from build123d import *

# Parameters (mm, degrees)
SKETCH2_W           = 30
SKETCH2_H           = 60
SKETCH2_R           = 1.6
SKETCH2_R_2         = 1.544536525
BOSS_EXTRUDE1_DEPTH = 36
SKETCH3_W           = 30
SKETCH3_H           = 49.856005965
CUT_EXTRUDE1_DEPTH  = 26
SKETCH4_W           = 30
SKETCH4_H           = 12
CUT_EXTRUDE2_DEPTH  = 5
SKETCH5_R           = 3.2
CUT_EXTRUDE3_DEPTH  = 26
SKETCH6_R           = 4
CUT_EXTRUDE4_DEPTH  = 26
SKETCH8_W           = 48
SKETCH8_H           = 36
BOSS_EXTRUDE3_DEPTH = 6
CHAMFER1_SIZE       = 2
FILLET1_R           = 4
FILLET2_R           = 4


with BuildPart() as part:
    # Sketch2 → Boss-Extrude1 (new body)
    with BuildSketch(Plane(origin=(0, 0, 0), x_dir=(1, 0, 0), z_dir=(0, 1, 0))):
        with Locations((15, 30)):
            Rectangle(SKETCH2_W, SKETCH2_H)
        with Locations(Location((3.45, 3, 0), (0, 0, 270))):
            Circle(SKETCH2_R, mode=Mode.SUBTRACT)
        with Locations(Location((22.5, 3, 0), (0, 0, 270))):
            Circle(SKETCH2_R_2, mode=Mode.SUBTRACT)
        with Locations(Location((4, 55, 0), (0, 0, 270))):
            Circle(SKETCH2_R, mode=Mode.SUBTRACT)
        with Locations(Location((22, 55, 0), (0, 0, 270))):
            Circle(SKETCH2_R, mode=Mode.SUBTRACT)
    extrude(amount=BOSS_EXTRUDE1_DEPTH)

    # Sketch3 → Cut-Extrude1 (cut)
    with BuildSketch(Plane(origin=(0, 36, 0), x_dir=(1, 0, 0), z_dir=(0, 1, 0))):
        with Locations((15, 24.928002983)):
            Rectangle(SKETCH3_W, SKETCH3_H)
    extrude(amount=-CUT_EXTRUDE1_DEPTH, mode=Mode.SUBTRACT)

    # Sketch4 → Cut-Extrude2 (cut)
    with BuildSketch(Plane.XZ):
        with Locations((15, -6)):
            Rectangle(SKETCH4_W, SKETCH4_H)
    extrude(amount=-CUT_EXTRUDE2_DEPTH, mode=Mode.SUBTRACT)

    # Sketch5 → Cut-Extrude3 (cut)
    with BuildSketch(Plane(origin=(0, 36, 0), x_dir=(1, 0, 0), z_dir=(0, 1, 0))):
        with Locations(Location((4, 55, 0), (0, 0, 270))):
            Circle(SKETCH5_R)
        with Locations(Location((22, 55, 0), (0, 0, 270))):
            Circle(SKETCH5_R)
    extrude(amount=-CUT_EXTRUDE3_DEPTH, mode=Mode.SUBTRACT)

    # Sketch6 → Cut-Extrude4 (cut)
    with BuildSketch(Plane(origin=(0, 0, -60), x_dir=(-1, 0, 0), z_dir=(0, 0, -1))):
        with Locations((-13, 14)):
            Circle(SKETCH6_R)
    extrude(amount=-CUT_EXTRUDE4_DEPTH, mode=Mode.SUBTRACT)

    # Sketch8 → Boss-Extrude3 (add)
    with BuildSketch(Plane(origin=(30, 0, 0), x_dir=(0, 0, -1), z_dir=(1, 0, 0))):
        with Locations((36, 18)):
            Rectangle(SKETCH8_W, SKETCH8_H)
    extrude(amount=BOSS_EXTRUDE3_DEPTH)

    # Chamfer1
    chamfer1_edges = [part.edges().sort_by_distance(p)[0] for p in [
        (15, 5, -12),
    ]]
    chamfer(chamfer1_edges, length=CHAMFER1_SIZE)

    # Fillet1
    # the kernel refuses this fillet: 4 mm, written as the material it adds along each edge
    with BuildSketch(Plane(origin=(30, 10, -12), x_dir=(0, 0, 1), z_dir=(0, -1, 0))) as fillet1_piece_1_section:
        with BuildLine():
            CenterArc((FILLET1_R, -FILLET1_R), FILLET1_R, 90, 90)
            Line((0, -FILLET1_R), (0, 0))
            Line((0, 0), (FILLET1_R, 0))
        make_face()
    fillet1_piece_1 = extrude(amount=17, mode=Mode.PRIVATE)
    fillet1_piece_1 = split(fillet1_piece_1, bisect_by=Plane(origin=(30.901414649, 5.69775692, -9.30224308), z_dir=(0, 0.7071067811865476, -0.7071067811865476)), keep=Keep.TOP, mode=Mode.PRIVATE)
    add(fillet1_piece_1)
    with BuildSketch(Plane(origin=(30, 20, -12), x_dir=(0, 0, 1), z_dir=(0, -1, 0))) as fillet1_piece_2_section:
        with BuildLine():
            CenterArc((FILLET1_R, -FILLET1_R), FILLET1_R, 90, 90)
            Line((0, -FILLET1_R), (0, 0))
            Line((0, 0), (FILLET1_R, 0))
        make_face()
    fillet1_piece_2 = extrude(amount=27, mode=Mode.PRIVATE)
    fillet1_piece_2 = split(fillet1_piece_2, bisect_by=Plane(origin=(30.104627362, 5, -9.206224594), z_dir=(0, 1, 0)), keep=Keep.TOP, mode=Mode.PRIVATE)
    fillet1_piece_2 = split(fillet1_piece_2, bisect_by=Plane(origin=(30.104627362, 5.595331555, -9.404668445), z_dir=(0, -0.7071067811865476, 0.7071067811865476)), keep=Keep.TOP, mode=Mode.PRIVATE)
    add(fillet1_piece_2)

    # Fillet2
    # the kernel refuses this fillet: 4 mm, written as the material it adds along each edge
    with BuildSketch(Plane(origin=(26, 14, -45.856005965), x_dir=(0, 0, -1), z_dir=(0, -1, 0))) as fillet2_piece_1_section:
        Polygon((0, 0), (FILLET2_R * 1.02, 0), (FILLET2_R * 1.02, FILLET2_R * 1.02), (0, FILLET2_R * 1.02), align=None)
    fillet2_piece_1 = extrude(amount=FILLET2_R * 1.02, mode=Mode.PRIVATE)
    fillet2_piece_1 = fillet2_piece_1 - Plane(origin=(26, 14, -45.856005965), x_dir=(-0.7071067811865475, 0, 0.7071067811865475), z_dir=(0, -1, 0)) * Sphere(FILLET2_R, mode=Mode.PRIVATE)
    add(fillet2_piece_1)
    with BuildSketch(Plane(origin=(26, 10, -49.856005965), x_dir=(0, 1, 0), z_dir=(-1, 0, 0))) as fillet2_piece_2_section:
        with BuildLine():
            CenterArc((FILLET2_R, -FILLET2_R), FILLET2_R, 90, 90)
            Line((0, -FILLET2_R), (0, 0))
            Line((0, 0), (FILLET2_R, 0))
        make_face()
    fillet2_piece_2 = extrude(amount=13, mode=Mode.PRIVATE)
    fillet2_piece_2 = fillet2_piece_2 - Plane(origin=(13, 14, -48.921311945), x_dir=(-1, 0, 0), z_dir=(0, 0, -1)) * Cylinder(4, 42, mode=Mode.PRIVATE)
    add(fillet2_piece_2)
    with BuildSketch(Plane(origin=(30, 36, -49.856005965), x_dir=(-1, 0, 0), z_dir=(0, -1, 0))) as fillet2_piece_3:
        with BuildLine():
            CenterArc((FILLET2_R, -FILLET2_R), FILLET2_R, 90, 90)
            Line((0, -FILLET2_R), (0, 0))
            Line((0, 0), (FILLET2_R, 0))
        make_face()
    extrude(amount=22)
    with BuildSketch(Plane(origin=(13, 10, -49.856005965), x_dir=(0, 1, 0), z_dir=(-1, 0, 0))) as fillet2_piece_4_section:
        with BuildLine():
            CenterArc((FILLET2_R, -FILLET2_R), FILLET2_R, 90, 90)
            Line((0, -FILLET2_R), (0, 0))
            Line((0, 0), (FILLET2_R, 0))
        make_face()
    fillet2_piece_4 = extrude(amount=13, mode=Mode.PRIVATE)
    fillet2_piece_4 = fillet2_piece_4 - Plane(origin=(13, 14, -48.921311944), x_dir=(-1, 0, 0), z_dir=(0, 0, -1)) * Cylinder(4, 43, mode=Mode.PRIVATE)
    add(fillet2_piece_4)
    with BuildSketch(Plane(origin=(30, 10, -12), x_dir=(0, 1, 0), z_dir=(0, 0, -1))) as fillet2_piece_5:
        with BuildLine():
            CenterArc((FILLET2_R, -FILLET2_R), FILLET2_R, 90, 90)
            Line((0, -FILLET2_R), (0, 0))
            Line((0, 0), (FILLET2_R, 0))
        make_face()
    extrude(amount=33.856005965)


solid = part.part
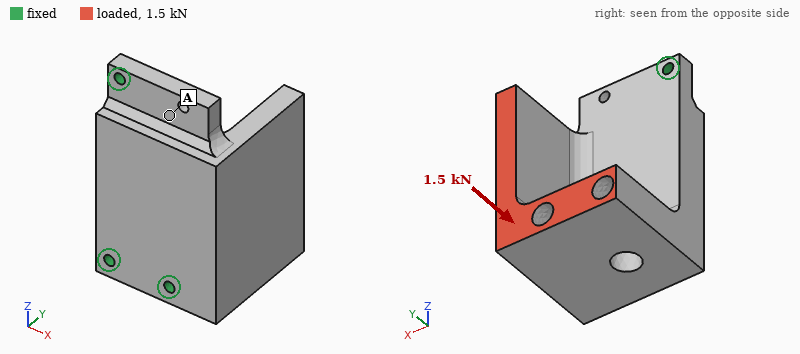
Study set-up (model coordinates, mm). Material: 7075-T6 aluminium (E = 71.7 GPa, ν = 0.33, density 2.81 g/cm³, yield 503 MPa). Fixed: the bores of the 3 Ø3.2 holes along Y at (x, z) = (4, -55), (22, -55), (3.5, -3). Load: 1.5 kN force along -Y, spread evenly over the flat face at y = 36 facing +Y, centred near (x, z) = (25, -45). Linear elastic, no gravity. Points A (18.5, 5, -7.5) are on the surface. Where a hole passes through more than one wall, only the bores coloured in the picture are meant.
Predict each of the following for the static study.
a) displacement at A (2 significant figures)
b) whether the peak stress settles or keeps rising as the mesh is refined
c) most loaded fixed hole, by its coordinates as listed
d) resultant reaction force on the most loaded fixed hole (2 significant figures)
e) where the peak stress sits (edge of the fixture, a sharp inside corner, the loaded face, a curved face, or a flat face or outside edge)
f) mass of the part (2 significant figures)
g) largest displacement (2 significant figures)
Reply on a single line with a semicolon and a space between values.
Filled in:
11 µm; keeps rising; (22, -55); 1.4 kN; edge of the fixture; 91 g; 31 µm
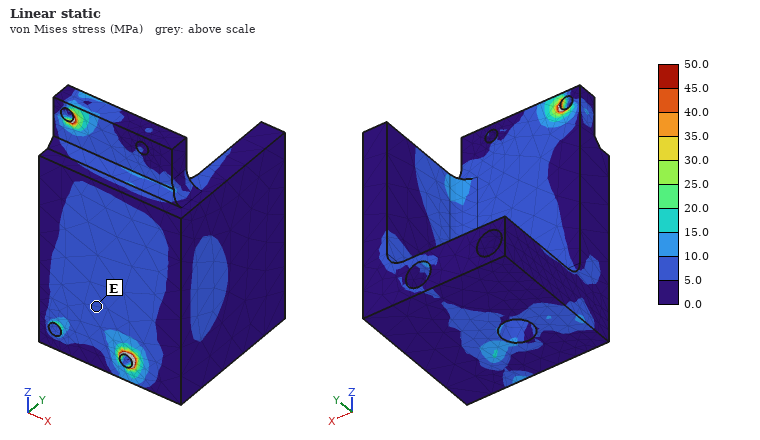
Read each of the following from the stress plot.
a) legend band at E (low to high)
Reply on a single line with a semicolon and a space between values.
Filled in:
5.0 to 10.0 MPa
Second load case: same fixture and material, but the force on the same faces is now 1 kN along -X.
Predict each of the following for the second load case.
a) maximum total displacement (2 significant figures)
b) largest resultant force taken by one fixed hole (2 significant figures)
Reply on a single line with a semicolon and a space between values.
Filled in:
59 µm; 1.2 kN
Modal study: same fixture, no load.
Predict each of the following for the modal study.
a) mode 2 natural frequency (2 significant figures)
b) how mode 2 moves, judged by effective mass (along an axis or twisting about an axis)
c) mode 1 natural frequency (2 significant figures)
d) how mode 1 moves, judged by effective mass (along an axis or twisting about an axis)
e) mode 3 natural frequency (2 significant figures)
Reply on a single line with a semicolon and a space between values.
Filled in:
7500 Hz; along X; 4500 Hz; along Y; 11 kHz
